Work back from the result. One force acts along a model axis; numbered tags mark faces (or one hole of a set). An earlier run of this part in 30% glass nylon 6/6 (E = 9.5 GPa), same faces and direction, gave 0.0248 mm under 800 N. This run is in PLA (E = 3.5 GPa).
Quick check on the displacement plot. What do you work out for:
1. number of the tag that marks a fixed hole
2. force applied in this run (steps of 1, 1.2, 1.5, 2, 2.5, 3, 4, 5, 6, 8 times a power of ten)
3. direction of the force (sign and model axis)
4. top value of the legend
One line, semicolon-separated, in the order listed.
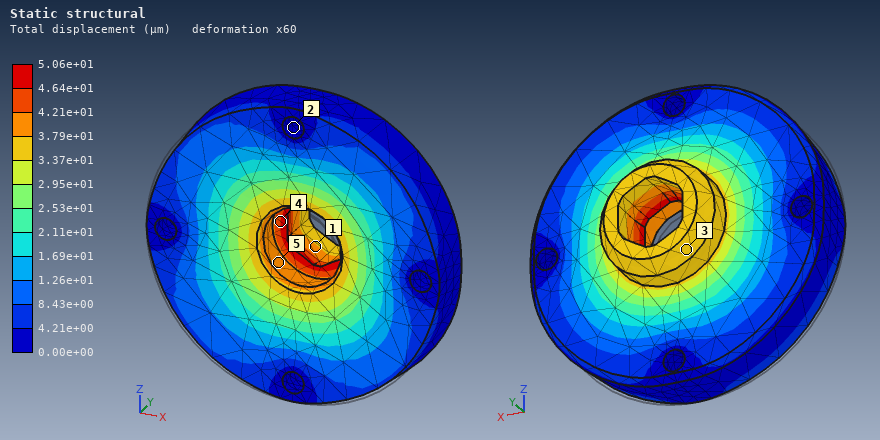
2; 600 N; +Y; 5.06e+01 µm
